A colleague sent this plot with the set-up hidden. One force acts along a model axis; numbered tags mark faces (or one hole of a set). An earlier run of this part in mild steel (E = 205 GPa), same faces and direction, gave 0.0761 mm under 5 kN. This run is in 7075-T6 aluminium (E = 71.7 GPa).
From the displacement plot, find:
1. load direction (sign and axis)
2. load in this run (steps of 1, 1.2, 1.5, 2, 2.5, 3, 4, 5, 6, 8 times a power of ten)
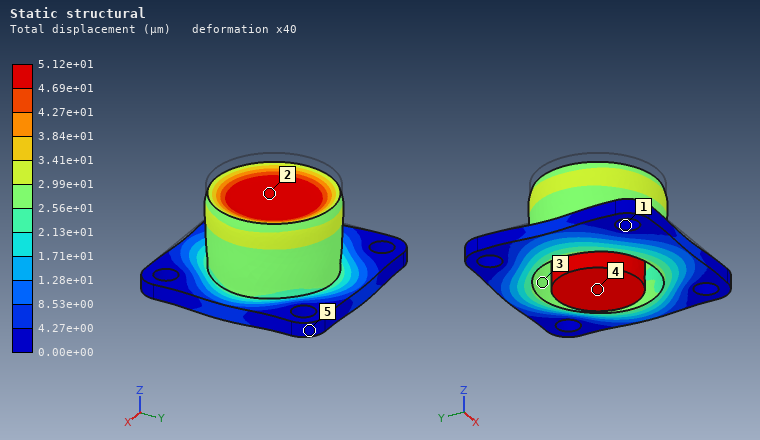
-Z
1.2 kN
